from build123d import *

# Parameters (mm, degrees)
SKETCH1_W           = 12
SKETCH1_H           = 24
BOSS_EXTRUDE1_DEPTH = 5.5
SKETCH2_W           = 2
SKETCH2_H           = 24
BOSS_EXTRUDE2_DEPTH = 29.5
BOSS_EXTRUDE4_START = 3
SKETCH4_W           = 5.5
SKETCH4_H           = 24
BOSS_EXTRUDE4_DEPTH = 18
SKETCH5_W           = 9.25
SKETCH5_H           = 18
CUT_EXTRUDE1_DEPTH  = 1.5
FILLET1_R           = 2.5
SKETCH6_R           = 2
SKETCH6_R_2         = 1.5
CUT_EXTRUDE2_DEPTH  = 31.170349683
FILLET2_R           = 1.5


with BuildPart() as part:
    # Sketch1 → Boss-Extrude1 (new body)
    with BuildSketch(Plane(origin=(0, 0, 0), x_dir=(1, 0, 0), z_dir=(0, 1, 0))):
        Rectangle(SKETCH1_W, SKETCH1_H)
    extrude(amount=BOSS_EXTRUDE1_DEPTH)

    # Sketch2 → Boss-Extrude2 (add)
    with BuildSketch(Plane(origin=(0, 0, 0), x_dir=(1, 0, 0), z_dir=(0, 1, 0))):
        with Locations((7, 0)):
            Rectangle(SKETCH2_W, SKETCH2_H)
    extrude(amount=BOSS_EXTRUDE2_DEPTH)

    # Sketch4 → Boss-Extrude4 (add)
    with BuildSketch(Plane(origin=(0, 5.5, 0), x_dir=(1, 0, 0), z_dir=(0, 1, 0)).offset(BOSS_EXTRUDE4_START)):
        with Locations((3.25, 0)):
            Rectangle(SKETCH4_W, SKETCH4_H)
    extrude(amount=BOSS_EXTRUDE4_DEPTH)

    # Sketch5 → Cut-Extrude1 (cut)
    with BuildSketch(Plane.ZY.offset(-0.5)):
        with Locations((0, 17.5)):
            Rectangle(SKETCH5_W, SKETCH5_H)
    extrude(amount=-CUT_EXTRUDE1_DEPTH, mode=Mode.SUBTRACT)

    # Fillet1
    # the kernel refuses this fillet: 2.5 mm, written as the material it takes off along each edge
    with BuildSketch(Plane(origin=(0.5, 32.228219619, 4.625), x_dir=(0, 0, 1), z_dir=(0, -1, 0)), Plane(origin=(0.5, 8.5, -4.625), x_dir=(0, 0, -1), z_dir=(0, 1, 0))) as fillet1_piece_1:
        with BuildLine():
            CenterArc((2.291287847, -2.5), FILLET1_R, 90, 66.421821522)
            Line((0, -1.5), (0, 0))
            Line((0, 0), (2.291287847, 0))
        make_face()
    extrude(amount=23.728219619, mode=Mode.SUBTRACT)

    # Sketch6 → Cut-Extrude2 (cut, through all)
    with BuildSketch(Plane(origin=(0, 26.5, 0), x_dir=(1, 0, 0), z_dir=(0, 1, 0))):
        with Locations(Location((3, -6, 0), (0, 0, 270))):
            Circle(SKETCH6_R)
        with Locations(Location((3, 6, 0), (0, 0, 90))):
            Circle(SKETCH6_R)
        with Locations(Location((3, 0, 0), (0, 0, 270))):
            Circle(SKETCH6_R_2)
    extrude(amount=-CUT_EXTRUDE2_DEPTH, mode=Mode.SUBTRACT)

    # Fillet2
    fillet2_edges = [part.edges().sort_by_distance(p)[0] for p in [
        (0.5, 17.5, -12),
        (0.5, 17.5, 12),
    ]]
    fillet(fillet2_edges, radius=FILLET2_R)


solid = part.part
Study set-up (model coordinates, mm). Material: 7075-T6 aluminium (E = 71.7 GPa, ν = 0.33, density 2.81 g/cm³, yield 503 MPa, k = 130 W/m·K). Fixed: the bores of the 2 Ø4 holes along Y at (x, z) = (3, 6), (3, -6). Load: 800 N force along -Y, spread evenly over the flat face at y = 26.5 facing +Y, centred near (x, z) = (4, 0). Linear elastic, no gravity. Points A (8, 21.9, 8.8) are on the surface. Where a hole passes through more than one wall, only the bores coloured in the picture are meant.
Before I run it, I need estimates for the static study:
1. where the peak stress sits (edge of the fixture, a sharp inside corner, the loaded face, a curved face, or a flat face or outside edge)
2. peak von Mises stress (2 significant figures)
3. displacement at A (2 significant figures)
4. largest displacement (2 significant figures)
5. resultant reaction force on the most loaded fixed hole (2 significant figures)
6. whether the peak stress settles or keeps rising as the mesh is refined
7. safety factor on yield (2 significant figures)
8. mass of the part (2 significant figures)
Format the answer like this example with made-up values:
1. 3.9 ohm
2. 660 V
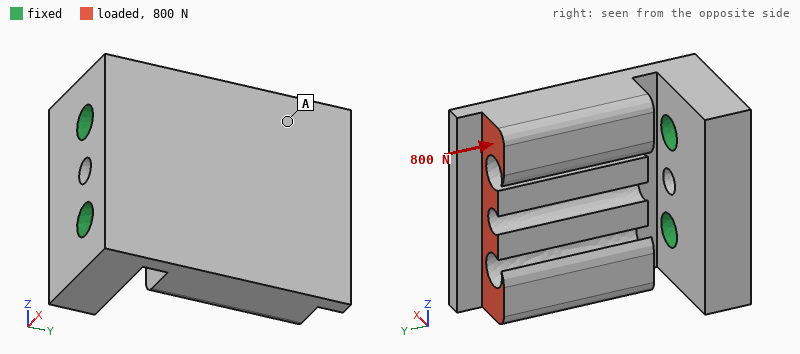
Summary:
1. a flat face or outside edge
2. 170 MPa
3. 0.16 mm
4. 0.24 mm
5. 400 N
6. settles
7. 2.9
8. 12 g
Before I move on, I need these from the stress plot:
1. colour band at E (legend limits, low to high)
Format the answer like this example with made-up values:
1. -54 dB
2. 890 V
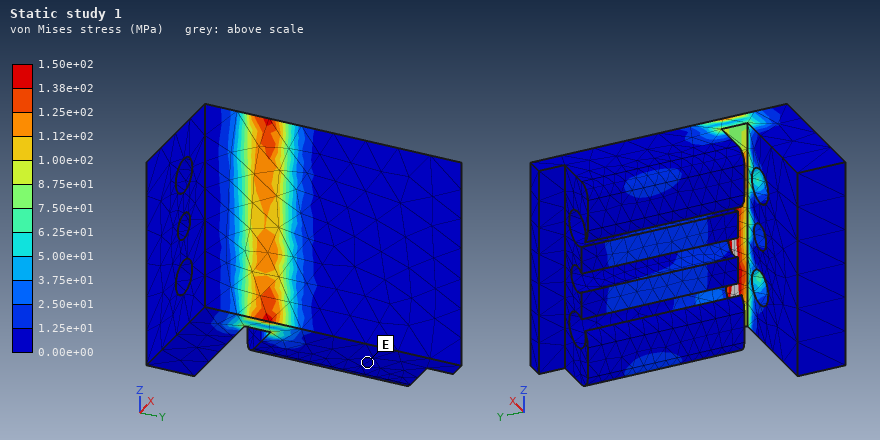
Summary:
1. 0.00e+00 to 1.25e+01 MPa
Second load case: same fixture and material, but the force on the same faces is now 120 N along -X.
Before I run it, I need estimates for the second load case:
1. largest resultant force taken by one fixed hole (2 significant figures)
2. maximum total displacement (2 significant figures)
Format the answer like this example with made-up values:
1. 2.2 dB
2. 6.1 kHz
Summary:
1. 61 N
2. 0.23 mm
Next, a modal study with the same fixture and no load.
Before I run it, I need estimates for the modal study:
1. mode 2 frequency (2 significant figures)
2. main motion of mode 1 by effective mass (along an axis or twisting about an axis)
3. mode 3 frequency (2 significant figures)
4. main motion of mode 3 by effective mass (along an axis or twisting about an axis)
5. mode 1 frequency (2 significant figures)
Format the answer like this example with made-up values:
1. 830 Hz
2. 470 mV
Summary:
1. 7900 Hz
2. along X
3. 11 kHz
4. along Z
5. 2200 Hz
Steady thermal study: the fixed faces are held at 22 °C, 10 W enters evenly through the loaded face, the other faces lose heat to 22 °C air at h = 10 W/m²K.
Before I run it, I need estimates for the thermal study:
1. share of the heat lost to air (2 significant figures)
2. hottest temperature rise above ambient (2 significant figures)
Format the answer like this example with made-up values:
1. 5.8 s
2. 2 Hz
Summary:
1. 3.0 %
2. 22 K
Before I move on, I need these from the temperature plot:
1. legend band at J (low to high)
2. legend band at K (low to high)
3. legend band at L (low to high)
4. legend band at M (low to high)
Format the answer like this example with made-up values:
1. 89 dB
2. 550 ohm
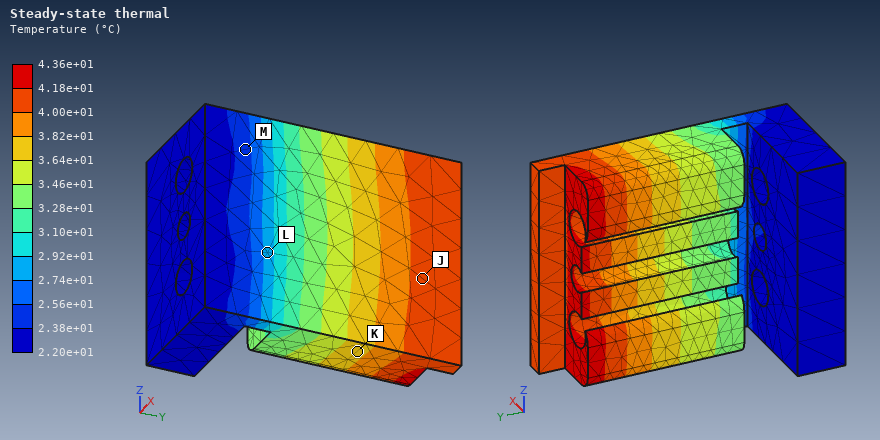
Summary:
1. 4.00e+01 to 4.18e+01 °C
2. 3.64e+01 to 3.82e+01 °C
3. 2.74e+01 to 2.92e+01 °C
4. 2.38e+01 to 2.56e+01 °C
